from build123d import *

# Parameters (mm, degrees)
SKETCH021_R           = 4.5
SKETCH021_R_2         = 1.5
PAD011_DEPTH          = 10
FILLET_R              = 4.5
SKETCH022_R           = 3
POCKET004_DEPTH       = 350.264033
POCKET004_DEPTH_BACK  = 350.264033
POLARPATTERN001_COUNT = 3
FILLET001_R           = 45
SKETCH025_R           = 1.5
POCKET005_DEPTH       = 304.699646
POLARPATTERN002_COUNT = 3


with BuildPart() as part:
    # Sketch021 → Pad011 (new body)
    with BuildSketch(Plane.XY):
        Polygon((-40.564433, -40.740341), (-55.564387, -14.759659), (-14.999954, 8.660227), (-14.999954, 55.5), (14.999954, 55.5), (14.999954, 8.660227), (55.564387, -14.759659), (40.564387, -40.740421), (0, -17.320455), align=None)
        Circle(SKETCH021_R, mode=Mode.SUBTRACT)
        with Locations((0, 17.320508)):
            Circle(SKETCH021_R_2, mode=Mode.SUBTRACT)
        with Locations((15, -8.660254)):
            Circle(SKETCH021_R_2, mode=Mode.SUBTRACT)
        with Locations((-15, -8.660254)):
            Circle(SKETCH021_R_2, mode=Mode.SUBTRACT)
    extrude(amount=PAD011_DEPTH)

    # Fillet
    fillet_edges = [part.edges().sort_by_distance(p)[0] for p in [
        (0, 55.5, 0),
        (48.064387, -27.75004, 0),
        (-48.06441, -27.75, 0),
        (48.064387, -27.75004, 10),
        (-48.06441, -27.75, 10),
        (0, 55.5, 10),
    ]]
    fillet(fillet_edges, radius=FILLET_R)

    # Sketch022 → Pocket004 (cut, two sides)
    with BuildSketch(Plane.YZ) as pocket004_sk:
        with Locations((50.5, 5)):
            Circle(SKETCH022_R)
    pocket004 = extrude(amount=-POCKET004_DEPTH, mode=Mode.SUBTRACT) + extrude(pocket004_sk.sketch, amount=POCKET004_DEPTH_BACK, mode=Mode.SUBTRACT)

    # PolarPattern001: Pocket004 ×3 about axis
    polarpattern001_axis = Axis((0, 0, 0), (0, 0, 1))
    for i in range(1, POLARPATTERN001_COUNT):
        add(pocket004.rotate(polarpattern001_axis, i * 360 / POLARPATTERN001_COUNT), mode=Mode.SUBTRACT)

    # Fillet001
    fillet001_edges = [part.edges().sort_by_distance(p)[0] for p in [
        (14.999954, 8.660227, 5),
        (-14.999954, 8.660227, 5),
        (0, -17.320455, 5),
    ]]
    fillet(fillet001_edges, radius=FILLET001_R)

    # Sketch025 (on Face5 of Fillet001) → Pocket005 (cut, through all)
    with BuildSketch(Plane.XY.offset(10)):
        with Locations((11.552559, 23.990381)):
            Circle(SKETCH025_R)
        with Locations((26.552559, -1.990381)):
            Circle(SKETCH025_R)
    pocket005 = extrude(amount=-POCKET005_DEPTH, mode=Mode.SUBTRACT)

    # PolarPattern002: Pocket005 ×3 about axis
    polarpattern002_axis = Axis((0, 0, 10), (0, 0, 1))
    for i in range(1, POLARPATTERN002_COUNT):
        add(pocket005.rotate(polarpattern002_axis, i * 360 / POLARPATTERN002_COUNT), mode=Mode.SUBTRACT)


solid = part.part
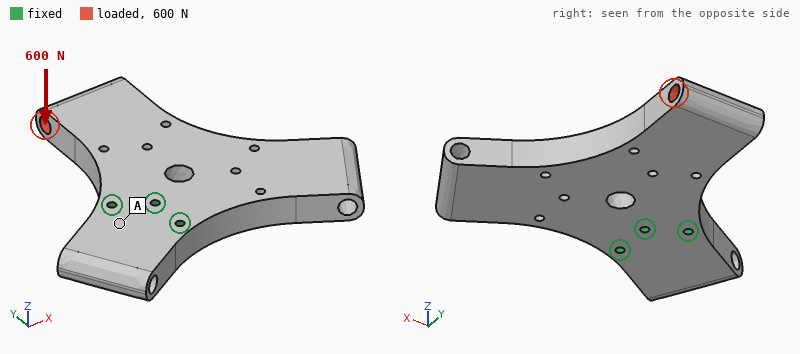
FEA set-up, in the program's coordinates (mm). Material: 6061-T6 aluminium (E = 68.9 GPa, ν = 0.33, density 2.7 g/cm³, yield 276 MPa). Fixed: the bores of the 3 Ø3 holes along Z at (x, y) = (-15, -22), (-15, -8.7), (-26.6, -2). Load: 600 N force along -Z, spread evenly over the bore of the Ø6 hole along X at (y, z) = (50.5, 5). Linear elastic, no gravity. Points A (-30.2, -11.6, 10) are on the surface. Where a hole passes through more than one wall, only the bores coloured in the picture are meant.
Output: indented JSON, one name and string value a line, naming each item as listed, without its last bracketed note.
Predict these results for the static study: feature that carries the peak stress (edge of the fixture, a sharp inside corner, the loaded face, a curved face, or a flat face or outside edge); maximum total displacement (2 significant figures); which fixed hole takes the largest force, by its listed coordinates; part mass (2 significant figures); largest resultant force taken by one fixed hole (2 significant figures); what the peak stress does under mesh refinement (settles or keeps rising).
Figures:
{
  "feature that carries the peak stress": "edge of the fixture",
  "maximum total displacement": "0.29 mm",
  "which fixed hole takes the largest force, by its listed coordinates": "(-15, -8.7)",
  "part mass": "120 g",
  "largest resultant force taken by one fixed hole": "1.0 kN",
  "what the peak stress does under mesh refinement": "keeps rising"
}
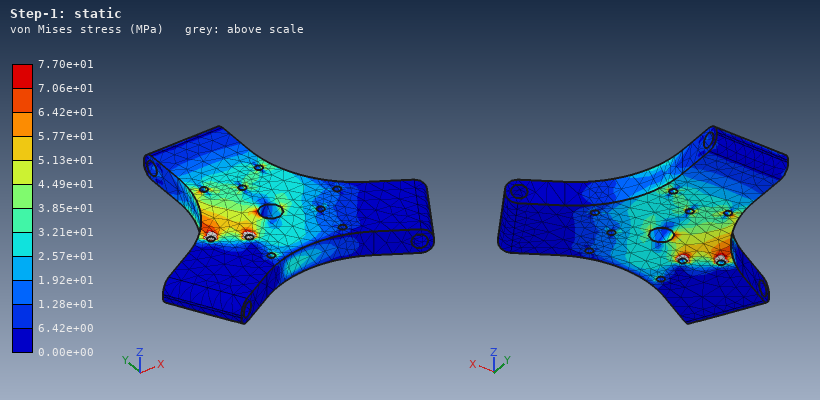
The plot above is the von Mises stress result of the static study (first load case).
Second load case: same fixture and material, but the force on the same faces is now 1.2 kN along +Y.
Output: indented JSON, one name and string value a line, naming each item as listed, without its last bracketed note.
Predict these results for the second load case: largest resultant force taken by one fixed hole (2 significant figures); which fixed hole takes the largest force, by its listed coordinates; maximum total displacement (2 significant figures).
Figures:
{
  "largest resultant force taken by one fixed hole": "1.0 kN",
  "which fixed hole takes the largest force, by its listed coordinates": "(-15, -8.7)",
  "maximum total displacement": "17 µm"
}
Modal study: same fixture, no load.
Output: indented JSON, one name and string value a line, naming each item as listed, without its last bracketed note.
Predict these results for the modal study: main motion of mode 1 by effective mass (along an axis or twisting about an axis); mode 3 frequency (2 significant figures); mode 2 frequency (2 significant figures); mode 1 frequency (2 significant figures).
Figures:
{
  "main motion of mode 1 by effective mass": "along Z",
  "mode 3 frequency": "4100 Hz",
  "mode 2 frequency": "2200 Hz",
  "mode 1 frequency": "1900 Hz"
}
